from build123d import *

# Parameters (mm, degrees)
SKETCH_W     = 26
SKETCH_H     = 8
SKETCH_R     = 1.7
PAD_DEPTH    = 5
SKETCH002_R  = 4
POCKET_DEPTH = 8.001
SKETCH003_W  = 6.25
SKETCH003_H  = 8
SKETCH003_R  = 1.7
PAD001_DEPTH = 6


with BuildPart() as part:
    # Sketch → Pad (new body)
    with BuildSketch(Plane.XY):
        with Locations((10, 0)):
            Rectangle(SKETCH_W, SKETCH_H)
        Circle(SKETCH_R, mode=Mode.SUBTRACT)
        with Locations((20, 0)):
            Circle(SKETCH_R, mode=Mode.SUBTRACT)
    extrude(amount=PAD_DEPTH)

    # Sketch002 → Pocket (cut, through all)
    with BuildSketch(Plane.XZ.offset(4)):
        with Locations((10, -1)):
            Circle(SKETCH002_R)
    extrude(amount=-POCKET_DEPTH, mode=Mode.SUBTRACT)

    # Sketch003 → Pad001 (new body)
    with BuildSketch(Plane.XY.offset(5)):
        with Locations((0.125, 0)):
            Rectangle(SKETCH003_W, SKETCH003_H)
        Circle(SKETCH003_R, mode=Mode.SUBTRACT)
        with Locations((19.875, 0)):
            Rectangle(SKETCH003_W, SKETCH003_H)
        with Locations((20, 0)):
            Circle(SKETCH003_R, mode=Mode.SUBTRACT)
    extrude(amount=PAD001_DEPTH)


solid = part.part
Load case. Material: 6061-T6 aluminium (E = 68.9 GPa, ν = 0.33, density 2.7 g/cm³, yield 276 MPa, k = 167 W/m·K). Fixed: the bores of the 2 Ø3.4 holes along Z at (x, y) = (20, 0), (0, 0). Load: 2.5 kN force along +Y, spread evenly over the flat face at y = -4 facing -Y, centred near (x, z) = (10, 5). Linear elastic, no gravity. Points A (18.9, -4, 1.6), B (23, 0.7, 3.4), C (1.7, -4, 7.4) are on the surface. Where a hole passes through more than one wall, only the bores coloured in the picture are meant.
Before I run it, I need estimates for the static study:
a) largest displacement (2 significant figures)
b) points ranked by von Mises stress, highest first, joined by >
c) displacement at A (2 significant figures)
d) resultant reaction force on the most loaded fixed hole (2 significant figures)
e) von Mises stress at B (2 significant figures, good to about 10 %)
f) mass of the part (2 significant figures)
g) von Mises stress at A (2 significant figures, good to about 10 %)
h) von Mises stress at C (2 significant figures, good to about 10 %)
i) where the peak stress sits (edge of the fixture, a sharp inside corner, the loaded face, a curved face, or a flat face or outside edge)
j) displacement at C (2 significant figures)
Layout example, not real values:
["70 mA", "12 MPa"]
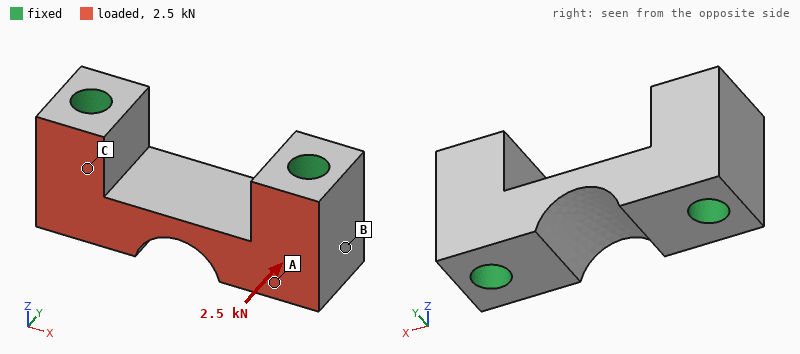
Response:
["5.3 µm", "A > C > B", "1.3 µm", "1.3 kN", "6.7 MPa", "3.5 g", "28 MPa", "17 MPa", "edge of the fixture", "0.91 µm"]
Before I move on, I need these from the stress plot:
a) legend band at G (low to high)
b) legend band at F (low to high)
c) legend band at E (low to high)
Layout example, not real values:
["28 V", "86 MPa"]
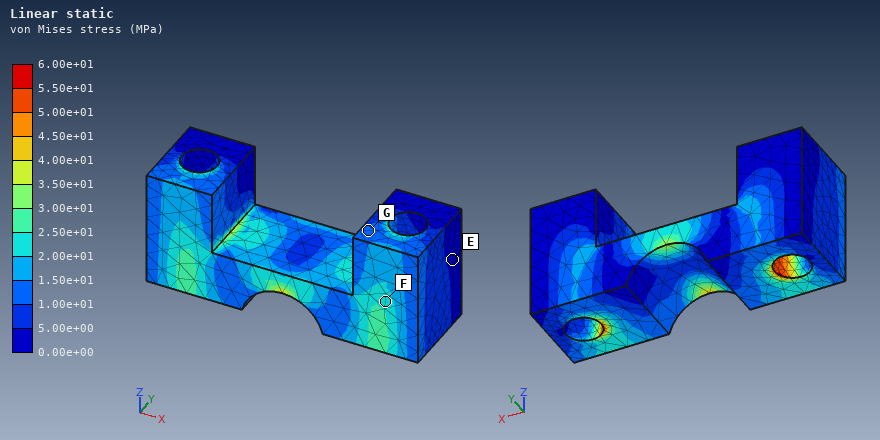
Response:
["1.00e+01 to 1.50e+01 MPa", "2.00e+01 to 2.50e+01 MPa", "0.00e+00 to 5.00e+00 MPa"]
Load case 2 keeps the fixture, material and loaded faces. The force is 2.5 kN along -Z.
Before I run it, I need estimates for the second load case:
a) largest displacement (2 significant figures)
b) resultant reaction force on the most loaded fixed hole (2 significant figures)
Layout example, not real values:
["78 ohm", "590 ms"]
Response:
["13 µm", "1.3 kN"]
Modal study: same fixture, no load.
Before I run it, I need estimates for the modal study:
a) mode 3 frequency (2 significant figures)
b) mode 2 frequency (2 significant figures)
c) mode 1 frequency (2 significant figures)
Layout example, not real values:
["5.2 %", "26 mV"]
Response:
["100 kHz", "70 kHz", "68 kHz"]
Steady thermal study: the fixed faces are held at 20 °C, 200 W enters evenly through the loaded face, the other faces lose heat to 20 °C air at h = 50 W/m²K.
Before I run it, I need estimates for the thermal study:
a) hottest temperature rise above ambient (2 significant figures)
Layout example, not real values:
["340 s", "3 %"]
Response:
["43 K"]
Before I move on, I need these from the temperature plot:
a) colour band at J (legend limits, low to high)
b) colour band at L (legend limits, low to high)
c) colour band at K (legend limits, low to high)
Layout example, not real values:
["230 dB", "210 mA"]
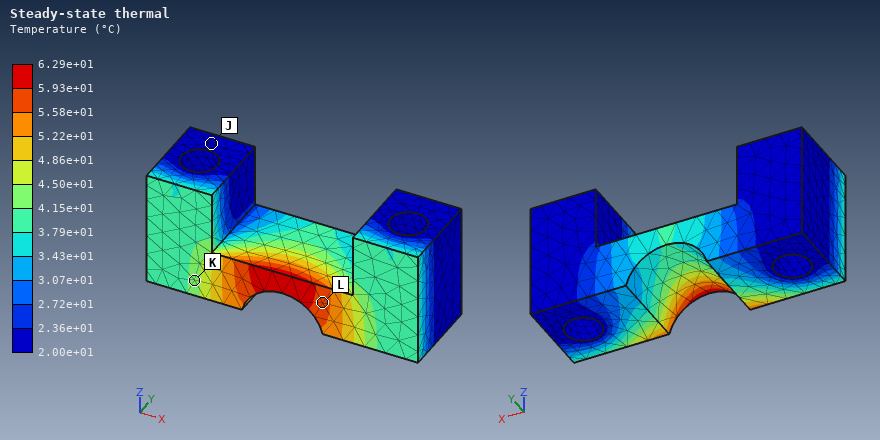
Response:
["2.00e+01 to 2.36e+01 °C", "5.58e+01 to 5.93e+01 °C", "4.15e+01 to 4.50e+01 °C"]
